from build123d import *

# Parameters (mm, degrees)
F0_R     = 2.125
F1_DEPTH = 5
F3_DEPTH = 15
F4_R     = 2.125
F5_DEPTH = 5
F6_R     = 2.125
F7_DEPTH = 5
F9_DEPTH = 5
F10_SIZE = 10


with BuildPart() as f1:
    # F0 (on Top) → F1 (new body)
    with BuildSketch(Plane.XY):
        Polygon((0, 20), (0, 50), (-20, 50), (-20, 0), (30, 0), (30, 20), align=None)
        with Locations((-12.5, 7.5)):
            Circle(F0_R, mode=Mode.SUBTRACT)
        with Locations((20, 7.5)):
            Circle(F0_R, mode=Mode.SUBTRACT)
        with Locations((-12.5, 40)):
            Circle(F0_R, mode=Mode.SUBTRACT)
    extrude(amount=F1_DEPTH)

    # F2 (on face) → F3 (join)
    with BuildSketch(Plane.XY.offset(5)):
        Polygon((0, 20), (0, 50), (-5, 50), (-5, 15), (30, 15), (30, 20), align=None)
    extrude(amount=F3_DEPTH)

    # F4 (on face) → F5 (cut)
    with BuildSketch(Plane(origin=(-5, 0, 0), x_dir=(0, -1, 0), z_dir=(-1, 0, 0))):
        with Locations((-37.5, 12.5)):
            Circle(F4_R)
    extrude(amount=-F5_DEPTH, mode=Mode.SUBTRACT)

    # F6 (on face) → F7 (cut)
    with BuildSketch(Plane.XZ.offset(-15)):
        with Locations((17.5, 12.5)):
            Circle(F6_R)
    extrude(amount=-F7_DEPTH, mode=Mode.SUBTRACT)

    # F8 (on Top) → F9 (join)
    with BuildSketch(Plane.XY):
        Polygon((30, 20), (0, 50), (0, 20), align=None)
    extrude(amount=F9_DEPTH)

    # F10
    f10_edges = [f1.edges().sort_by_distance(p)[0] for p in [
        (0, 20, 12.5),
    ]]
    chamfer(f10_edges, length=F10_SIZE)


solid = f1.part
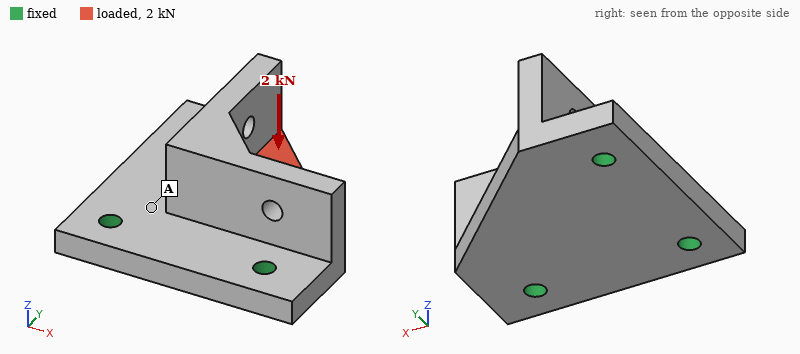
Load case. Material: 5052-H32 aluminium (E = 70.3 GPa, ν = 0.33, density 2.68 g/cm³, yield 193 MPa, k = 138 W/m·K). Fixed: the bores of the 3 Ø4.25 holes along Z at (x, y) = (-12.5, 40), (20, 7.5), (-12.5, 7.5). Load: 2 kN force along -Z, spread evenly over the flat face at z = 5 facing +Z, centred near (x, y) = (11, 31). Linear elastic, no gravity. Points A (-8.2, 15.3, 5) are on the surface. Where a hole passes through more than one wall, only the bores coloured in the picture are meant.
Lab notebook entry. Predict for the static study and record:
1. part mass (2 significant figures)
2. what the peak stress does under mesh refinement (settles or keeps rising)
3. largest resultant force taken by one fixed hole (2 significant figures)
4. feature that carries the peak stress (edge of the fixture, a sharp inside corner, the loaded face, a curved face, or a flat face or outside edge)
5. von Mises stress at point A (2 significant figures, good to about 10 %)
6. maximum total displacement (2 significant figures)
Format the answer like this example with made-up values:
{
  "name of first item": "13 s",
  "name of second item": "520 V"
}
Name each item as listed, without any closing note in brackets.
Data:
{
  "part mass": "42 g",
  "what the peak stress does under mesh refinement": "keeps rising",
  "largest resultant force taken by one fixed hole": "1.2 kN",
  "feature that carries the peak stress": "edge of the fixture",
  "von Mises stress at point A": "20 MPa",
  "maximum total displacement": "81 µm"
}
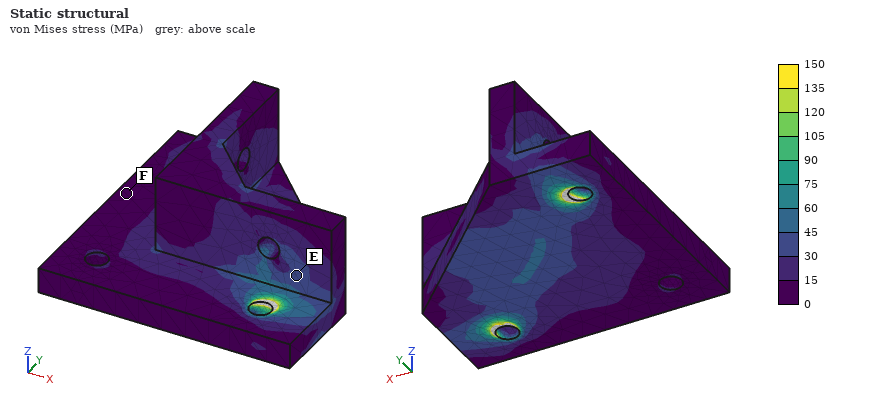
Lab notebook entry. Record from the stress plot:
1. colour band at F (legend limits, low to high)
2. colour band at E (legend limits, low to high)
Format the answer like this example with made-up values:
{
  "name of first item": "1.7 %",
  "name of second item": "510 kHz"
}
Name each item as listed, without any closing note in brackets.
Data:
{
  "colour band at F": "0 to 15 MPa",
  "colour band at E": "30 to 45 MPa"
}
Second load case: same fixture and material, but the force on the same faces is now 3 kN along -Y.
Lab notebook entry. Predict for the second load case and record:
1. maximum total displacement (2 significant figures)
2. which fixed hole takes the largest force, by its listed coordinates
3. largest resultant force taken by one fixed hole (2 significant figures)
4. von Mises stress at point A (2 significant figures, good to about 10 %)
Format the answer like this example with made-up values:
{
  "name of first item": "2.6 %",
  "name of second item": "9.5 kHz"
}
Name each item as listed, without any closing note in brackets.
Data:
{
  "maximum total displacement": "22 µm",
  "which fixed hole takes the largest force, by its listed coordinates": "(20, 7.5)",
  "largest resultant force taken by one fixed hole": "1.6 kN",
  "von Mises stress at point A": "20 MPa"
}
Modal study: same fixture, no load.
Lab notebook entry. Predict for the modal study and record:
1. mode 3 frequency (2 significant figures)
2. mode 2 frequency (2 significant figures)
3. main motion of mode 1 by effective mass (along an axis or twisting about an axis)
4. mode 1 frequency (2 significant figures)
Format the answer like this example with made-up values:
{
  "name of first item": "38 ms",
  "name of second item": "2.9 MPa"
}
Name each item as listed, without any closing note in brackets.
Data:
{
  "mode 3 frequency": "14 kHz",
  "mode 2 frequency": "13 kHz",
  "main motion of mode 1 by effective mass": "along Z",
  "mode 1 frequency": "8400 Hz"
}
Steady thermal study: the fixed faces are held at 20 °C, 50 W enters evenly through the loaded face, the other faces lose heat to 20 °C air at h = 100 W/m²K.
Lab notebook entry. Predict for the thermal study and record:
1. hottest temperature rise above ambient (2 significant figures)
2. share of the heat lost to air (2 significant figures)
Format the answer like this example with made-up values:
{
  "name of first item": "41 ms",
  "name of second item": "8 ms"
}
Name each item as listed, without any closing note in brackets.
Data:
{
  "hottest temperature rise above ambient": "28 K",
  "share of the heat lost to air": "12 %"
}
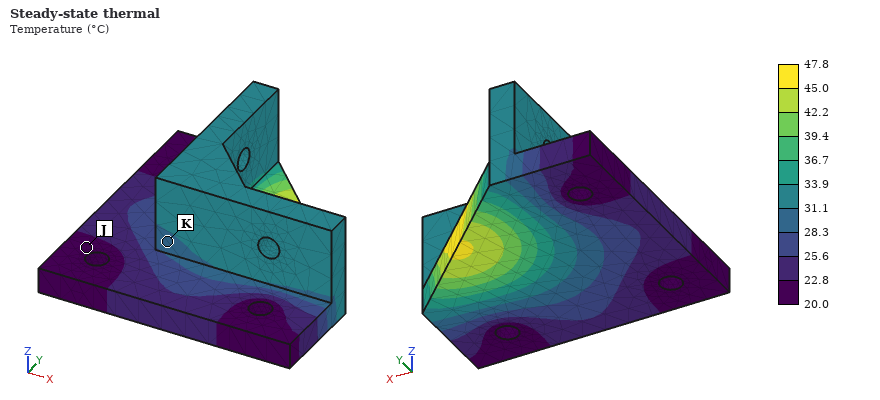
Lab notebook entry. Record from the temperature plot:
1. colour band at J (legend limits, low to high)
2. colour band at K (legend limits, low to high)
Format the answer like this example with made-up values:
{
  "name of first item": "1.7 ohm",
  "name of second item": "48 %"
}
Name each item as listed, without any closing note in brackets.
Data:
{
  "colour band at J": "20.0 to 22.8 °C",
  "colour band at K": "28.3 to 31.1 °C"
}
